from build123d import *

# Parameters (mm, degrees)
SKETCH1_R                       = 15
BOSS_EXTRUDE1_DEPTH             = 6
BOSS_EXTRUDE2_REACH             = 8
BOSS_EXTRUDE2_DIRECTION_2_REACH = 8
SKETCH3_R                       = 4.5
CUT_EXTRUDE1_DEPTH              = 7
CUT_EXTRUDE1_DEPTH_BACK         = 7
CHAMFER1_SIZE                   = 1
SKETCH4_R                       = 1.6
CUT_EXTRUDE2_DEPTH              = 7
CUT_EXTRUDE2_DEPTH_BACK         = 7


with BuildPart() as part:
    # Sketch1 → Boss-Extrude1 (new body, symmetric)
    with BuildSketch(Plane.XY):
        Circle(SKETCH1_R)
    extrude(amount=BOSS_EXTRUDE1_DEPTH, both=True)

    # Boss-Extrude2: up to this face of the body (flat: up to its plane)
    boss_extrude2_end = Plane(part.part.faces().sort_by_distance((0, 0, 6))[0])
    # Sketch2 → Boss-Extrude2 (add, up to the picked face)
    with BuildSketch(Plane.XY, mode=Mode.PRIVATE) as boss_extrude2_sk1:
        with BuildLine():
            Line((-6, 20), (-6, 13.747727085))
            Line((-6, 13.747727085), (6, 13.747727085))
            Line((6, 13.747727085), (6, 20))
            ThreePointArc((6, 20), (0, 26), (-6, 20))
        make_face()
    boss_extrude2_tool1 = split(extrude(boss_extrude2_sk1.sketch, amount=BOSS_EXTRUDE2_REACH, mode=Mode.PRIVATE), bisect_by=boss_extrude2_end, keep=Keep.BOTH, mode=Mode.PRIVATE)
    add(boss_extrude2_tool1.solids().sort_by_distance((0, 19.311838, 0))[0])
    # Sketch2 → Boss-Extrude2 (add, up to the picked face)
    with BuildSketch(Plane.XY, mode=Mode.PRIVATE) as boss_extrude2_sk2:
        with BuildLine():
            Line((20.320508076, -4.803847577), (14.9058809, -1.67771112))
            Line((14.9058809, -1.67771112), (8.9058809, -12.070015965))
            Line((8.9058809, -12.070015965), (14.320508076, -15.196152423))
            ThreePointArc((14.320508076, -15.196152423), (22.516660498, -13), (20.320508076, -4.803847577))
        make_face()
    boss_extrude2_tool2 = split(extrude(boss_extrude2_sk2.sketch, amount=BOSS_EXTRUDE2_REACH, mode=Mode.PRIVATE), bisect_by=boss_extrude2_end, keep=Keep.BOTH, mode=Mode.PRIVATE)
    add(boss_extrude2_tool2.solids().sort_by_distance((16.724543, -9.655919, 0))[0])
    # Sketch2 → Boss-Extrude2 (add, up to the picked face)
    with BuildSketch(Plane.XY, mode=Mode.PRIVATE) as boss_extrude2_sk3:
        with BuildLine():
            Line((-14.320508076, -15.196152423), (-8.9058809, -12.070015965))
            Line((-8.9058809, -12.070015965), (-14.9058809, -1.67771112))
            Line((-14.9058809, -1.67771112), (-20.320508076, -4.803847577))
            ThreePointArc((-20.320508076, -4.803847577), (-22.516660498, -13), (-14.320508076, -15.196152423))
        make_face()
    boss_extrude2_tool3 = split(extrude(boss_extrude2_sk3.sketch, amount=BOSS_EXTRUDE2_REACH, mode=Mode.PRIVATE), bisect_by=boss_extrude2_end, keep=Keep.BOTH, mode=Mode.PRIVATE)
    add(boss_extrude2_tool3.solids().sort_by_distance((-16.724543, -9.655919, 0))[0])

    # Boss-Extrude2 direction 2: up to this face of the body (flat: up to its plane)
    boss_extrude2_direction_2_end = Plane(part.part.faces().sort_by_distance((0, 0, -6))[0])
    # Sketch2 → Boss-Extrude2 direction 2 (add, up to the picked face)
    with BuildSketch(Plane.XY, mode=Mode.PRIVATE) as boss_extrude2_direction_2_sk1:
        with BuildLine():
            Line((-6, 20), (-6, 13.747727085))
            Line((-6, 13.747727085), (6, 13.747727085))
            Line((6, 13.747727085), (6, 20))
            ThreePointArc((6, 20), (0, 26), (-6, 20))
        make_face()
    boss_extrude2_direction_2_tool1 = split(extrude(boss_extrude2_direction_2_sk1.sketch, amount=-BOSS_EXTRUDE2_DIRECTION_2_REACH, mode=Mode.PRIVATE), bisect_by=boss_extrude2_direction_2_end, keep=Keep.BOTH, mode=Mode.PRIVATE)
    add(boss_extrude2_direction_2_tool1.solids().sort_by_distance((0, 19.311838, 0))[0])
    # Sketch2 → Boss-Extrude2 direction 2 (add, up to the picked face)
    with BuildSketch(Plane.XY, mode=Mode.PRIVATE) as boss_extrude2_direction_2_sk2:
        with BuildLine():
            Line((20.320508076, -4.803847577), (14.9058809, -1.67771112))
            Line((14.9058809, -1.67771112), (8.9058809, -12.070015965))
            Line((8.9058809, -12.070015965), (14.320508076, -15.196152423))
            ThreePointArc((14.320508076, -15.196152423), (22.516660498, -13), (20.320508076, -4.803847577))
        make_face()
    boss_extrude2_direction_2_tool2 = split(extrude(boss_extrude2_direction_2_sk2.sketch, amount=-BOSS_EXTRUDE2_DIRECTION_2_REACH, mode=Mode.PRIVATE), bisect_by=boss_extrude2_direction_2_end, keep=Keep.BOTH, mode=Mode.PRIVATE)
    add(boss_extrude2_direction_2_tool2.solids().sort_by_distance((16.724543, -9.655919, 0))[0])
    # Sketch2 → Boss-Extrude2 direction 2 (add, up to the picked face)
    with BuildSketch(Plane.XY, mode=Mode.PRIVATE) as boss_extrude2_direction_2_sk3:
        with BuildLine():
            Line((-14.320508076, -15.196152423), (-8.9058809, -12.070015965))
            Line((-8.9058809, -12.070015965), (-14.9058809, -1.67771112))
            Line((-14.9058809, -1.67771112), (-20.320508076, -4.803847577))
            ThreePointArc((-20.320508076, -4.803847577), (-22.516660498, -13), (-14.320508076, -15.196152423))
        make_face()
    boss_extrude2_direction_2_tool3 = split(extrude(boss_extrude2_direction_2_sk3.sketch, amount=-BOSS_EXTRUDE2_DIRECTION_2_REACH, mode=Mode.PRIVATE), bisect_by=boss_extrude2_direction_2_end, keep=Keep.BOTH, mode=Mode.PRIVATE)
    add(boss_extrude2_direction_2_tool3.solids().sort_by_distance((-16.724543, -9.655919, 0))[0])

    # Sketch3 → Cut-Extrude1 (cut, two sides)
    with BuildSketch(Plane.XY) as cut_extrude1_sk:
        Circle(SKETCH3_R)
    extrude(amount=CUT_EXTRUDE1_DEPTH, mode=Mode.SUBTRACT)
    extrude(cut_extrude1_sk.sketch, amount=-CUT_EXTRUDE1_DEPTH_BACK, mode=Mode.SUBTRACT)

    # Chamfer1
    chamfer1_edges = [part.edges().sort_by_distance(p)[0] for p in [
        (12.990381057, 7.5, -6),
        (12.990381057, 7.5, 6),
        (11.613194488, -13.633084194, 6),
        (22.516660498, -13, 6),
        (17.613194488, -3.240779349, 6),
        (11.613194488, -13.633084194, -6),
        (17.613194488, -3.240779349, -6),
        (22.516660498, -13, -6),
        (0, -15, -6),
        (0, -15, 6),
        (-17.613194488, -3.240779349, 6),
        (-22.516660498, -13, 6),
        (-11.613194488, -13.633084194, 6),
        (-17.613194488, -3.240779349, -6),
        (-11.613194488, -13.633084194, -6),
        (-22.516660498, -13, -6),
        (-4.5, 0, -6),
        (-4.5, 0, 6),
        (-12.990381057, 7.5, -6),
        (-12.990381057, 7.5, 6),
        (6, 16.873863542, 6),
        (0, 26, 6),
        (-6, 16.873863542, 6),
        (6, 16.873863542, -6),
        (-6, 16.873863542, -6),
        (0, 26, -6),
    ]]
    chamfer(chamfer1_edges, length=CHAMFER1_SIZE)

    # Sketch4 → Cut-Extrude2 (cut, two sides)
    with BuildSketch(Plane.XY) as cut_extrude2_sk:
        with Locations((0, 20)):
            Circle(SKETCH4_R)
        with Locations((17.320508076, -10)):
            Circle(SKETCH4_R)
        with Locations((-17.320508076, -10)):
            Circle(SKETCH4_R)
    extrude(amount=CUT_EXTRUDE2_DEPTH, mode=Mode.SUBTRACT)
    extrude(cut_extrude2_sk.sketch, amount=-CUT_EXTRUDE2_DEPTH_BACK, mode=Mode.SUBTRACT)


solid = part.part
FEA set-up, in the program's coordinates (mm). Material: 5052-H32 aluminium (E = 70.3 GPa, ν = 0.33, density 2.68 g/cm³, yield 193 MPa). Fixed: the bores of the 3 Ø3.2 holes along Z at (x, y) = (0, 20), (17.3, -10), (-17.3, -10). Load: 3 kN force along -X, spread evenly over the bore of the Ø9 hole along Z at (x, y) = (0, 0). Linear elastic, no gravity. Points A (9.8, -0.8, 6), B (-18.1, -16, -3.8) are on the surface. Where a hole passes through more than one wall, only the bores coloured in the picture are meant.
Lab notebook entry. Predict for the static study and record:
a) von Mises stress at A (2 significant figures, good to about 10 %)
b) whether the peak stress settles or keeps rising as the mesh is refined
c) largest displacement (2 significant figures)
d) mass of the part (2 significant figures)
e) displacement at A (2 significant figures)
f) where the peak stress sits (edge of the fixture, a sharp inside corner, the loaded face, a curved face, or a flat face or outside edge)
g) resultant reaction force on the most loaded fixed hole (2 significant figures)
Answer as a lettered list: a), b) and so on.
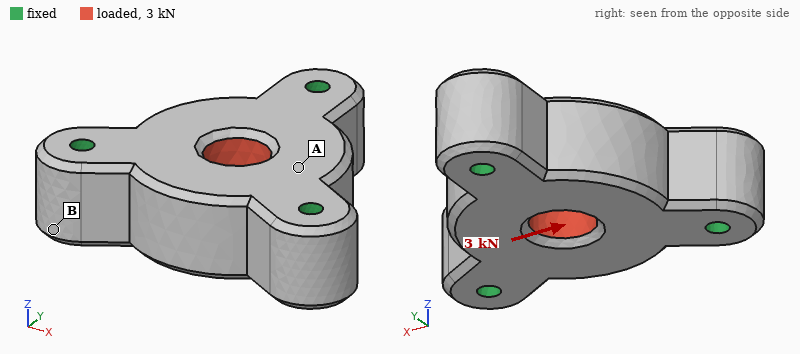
a) 11 MPa
b) keeps rising
c) 4.7 µm
d) 31 g
e) 2.9 µm
f) edge of the fixture
g) 1.3 kN
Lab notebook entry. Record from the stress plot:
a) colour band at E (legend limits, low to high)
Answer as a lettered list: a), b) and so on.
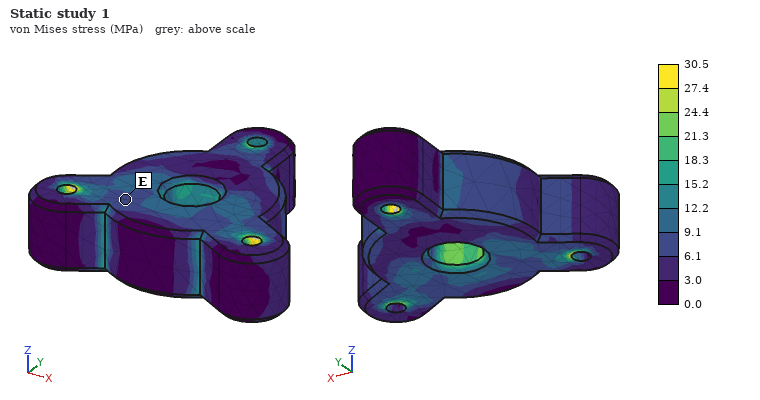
a) 6.1 to 9.1 MPa
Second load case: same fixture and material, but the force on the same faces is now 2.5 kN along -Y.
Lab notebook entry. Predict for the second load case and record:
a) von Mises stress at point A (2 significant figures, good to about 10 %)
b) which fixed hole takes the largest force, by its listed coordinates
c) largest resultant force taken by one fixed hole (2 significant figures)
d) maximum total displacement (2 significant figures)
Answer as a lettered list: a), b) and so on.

a) 3.4 MPa
b) (0, 20)
c) 1.2 kN
d) 4.0 µm
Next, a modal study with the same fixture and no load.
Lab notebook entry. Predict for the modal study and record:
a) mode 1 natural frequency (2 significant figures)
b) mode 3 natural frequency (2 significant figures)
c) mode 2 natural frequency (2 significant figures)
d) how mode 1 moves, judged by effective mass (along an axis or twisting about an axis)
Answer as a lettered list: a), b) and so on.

a) 28 kHz
b) 35 kHz
c) 35 kHz
d) along Z
